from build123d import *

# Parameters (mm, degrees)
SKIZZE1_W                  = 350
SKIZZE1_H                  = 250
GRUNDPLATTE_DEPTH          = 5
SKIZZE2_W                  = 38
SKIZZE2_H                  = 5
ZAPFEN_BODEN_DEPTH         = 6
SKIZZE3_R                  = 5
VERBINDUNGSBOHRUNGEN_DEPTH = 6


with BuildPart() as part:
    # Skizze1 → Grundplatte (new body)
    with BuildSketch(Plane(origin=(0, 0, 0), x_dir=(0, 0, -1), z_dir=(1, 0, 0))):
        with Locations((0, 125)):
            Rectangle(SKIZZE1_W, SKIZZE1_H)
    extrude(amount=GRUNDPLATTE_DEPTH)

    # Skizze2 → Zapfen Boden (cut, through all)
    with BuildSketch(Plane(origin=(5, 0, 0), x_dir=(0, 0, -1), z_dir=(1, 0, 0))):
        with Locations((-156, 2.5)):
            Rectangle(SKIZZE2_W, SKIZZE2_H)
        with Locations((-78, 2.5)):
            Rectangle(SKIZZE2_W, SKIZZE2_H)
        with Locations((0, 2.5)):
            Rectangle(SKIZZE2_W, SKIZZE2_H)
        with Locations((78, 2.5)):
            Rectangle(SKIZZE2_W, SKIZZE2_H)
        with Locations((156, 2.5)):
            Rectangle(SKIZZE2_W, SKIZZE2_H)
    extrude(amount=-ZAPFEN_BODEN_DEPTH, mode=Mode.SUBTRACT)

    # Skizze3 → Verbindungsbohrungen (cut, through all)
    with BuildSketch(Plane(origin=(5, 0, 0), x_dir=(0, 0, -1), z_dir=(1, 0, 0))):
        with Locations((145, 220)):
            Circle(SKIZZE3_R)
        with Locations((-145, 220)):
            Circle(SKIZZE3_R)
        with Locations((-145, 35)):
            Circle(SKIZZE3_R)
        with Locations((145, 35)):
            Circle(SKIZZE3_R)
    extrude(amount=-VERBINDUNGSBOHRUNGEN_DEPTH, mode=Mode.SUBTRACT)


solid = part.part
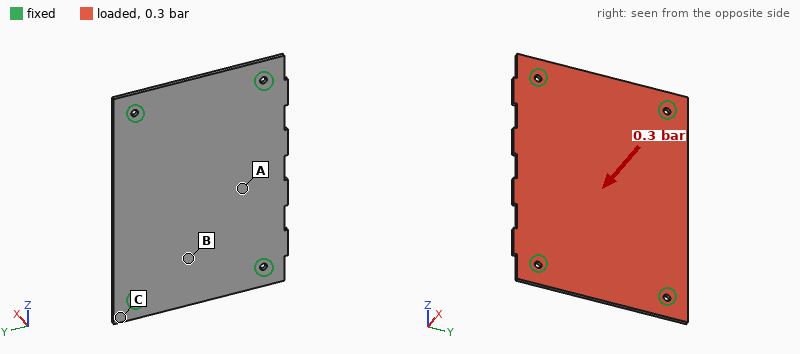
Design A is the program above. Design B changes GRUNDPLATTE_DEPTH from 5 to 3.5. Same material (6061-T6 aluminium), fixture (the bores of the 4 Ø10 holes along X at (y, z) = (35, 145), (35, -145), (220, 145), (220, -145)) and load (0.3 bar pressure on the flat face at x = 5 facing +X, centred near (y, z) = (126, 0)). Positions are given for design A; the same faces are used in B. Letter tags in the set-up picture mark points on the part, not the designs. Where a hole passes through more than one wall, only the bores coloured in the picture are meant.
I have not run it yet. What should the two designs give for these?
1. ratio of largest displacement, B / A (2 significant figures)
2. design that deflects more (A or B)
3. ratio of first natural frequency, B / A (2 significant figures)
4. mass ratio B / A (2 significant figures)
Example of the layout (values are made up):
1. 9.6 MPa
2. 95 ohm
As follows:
1. 2.9
2. B
3. 0.71
4. 0.70
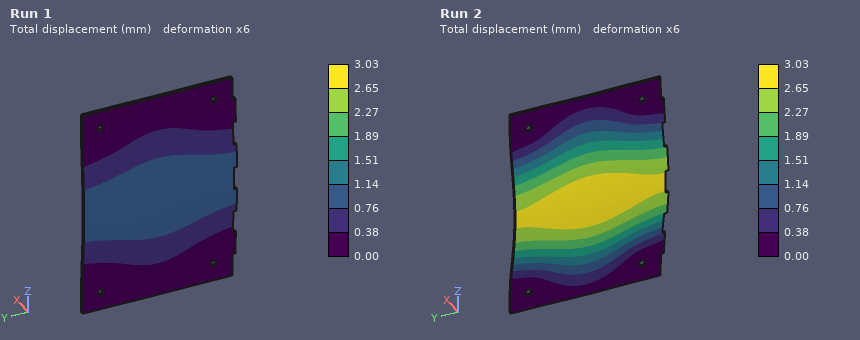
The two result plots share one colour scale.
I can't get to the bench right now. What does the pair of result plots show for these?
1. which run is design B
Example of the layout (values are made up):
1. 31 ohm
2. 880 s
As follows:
1. Run 2
